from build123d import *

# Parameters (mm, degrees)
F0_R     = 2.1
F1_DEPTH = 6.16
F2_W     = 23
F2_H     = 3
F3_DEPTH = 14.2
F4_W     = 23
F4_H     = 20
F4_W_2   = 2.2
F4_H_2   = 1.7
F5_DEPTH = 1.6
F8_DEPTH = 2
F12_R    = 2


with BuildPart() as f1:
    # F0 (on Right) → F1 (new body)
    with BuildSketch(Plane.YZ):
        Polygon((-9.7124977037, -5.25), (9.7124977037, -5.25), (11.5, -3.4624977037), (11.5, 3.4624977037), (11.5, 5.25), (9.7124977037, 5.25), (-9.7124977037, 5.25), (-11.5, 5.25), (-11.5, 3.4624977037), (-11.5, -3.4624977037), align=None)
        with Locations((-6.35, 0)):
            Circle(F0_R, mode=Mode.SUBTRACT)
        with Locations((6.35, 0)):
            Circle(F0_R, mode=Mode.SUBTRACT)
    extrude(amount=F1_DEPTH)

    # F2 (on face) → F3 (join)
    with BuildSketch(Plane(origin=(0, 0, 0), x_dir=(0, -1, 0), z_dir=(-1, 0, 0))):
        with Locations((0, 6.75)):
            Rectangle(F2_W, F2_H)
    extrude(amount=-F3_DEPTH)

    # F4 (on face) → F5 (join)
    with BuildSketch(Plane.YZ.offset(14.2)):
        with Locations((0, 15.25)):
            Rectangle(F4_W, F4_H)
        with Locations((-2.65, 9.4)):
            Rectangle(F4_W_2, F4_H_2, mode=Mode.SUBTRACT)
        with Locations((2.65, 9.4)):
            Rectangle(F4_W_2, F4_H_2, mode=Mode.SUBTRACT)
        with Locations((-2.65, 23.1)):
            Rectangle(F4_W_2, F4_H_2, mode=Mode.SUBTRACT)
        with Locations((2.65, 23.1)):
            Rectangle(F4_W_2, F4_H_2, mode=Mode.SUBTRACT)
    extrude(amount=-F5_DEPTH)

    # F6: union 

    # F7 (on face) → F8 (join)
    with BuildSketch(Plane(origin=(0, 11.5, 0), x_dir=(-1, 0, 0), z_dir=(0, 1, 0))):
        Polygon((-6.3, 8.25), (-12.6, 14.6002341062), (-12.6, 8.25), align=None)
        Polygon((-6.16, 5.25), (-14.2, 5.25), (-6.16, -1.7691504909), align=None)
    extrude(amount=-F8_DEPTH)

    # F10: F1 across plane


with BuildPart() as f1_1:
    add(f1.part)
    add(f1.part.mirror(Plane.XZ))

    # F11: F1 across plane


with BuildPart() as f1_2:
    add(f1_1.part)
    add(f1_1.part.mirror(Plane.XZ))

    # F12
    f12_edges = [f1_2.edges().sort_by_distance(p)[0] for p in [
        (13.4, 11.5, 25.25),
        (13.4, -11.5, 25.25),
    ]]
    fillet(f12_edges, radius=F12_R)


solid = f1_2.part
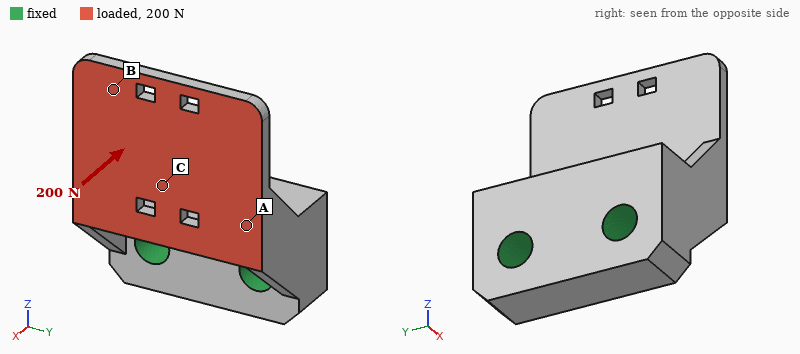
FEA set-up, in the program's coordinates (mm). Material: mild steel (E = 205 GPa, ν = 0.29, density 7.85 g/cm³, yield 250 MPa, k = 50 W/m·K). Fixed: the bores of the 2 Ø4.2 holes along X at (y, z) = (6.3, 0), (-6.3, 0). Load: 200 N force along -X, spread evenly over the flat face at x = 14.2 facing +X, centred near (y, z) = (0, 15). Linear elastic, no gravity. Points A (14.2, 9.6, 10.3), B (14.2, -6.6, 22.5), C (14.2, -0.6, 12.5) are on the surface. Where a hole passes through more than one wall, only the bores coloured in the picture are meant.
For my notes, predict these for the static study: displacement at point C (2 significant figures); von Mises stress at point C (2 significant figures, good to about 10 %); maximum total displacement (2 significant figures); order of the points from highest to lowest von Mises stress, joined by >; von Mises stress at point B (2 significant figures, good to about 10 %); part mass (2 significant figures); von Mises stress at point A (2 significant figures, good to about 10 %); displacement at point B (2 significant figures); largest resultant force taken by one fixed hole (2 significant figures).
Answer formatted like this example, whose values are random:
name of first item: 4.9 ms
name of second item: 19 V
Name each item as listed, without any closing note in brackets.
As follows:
displacement at point C: 9.8 µm
von Mises stress at point C: 32 MPa
maximum total displacement: 49 µm
order of the points from highest to lowest von Mises stress, joined by >: A > C > B
von Mises stress at point B: 15 MPa
part mass: 24 g
von Mises stress at point A: 51 MPa
displacement at point B: 36 µm
largest resultant force taken by one fixed hole: 100 N
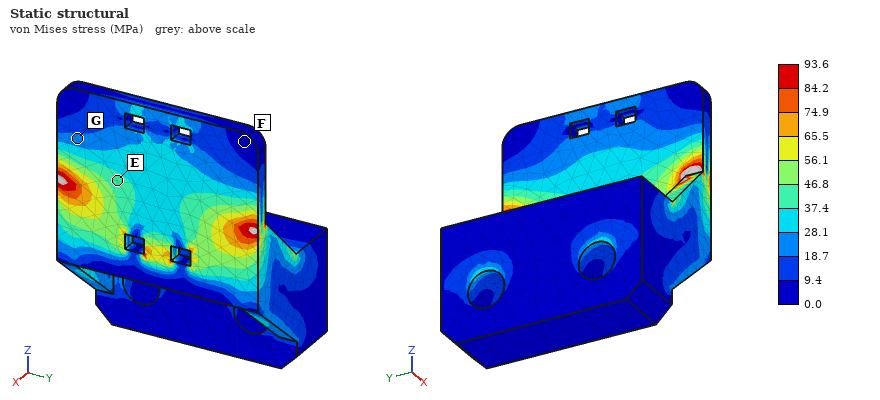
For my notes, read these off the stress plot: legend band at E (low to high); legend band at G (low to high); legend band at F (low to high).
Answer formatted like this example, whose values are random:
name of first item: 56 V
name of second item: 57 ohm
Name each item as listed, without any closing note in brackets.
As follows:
legend band at E: 37.4 to 46.8 MPa
legend band at G: 18.7 to 28.1 MPa
legend band at F: 0.0 to 9.4 MPa
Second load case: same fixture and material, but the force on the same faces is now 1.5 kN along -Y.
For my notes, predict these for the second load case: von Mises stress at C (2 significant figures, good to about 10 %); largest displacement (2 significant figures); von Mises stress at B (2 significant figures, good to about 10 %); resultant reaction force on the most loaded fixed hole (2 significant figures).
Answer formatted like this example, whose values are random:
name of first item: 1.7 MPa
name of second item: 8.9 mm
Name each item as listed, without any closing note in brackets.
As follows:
von Mises stress at C: 26 MPa
largest displacement: 24 µm
von Mises stress at B: 27 MPa
resultant reaction force on the most loaded fixed hole: 1.7 kN
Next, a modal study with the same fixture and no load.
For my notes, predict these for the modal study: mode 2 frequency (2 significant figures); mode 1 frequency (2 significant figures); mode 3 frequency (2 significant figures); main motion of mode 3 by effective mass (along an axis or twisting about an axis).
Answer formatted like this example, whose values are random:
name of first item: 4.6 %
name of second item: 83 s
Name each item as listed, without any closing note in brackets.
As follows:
mode 2 frequency: 11 kHz
mode 1 frequency: 5600 Hz
mode 3 frequency: 17 kHz
main motion of mode 3 by effective mass: along Z
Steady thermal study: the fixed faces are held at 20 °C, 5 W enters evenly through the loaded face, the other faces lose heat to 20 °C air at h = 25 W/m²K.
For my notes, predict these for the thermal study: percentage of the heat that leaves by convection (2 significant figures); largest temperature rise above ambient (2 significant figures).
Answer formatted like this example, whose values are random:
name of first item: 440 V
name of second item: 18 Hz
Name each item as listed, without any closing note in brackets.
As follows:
percentage of the heat that leaves by convection: 8.9 %
largest temperature rise above ambient: 30 K
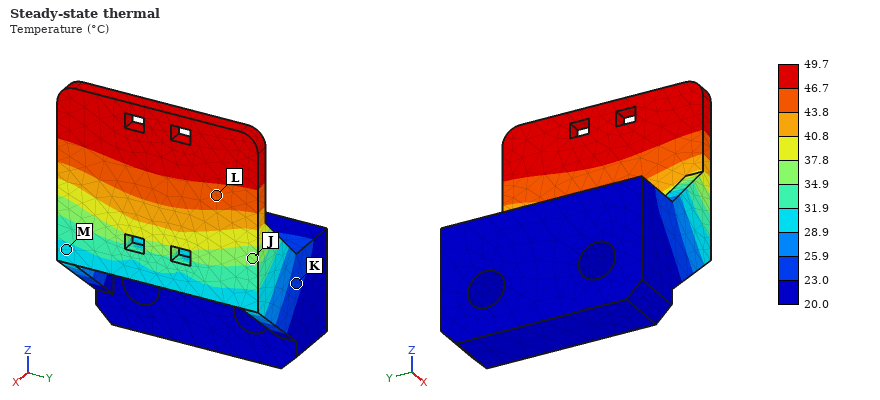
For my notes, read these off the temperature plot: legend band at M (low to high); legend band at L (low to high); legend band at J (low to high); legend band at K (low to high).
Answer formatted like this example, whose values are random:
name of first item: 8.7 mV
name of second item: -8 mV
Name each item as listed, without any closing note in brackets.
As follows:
legend band at M: 28.9 to 31.9 °C
legend band at L: 43.8 to 46.7 °C
legend band at J: 34.9 to 37.8 °C
legend band at K: 23.0 to 25.9 °C
